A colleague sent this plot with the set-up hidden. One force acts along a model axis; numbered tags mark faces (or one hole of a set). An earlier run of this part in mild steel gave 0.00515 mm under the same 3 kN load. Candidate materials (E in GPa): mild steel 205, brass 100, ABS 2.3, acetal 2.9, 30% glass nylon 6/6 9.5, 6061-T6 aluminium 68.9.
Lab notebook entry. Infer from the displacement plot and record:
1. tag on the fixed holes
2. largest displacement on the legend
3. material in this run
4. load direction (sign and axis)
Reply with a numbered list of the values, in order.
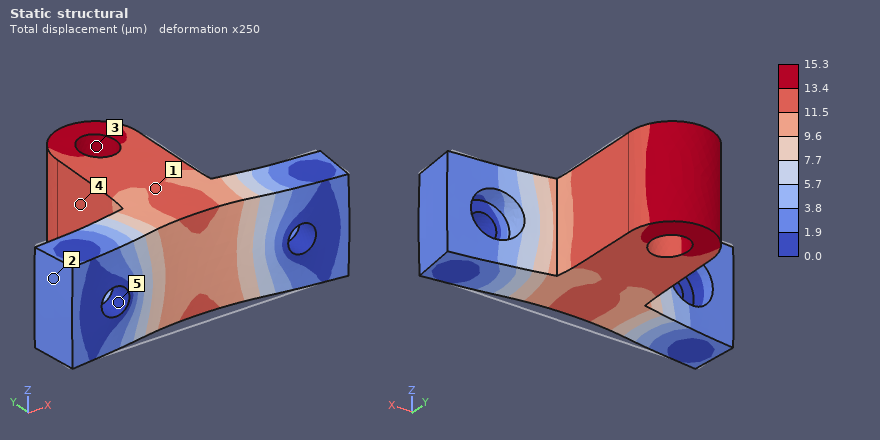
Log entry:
1. 5
2. 15.3 µm
3. 6061-T6 aluminium
4. +Y
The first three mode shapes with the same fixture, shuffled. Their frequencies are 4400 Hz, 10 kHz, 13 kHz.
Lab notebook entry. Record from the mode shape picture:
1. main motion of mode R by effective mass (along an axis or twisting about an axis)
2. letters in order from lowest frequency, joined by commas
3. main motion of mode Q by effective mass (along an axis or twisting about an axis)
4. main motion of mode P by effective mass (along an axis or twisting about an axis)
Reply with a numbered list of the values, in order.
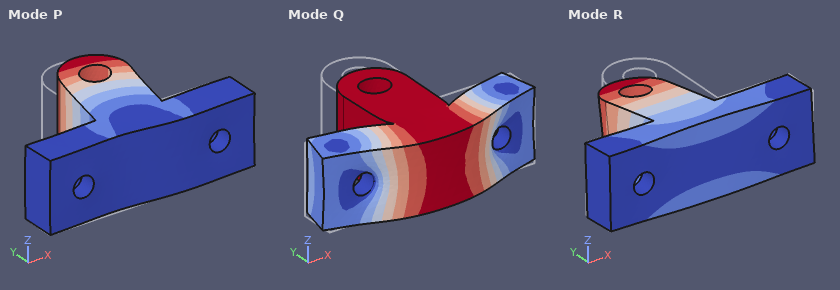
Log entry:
1. along Z
2. R, P, Q
3. along Y
4. along X
